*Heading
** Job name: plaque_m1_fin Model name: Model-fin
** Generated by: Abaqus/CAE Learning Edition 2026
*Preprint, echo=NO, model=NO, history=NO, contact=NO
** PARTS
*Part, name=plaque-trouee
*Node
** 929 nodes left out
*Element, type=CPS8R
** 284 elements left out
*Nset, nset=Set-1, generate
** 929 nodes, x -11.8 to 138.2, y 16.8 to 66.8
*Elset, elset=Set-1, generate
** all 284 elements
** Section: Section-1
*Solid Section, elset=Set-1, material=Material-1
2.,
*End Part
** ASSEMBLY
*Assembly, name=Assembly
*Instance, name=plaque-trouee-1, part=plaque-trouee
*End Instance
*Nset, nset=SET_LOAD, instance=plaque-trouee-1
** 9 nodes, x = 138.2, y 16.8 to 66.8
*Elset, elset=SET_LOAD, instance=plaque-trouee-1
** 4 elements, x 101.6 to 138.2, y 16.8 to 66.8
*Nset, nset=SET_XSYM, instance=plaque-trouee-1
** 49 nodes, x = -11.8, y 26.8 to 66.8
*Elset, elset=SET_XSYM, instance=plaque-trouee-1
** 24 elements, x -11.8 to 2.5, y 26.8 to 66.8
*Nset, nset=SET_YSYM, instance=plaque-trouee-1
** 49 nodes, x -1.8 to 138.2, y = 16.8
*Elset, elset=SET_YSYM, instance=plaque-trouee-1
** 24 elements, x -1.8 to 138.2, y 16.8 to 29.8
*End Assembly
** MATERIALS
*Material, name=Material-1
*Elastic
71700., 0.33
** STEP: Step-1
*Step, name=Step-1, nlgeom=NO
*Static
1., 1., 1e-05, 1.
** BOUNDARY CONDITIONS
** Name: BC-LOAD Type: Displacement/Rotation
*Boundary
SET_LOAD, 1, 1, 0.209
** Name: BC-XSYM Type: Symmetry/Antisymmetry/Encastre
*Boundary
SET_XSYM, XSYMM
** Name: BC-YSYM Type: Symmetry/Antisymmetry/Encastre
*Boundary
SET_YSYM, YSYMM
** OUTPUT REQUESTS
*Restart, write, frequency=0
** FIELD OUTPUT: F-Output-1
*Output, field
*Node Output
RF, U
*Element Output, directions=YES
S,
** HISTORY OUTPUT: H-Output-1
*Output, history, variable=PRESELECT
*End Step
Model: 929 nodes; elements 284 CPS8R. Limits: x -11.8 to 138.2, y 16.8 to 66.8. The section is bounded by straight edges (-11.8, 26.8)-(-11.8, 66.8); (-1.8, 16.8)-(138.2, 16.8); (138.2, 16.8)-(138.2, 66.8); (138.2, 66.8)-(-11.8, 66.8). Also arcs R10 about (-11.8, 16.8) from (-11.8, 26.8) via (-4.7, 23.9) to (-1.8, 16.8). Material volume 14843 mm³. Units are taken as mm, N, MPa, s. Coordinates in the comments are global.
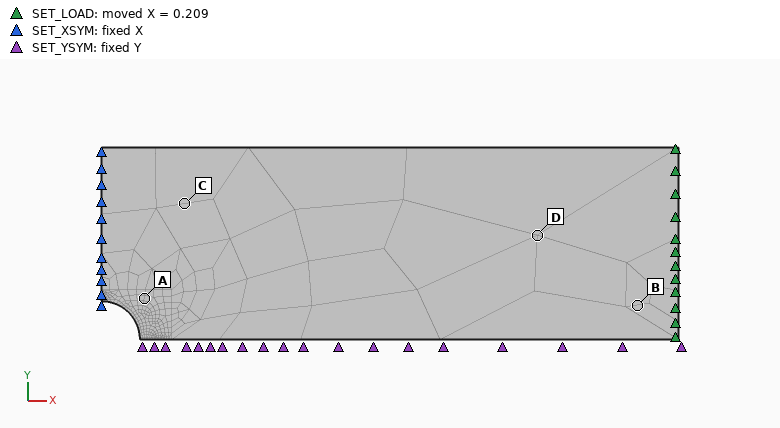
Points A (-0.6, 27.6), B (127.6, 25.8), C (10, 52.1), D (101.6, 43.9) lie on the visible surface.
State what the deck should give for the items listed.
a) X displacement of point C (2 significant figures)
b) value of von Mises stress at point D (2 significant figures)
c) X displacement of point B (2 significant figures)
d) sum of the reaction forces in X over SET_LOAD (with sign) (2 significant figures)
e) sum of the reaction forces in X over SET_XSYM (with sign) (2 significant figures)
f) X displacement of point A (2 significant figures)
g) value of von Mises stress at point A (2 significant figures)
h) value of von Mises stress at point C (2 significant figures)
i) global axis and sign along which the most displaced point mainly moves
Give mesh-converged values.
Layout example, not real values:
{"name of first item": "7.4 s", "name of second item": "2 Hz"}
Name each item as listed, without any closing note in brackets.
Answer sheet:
{"X displacement of point C": "0.032 mm", "value of von Mises stress at point D": "97 MPa", "X displacement of point B": "0.19 mm", "sum of the reaction forces in X over SET_LOAD (with sign)": "9700 N", "sum of the reaction forces in X over SET_XSYM (with sign)": "-9700 N", "X displacement of point A": "0.027 mm", "value of von Mises stress at point A": "130 MPa", "value of von Mises stress at point C": "110 MPa", "global axis and sign along which the most displaced point mainly moves": "+X"}
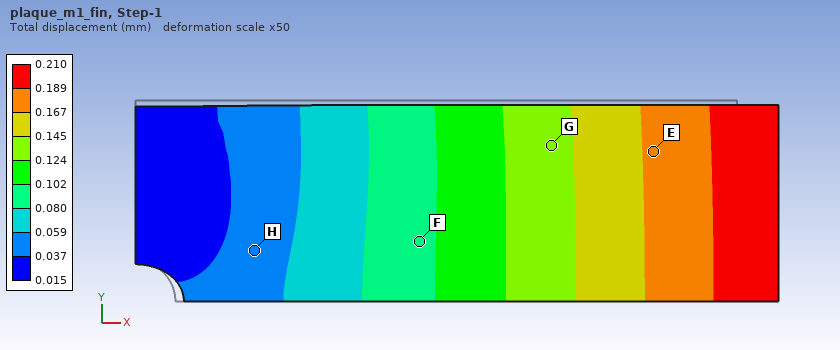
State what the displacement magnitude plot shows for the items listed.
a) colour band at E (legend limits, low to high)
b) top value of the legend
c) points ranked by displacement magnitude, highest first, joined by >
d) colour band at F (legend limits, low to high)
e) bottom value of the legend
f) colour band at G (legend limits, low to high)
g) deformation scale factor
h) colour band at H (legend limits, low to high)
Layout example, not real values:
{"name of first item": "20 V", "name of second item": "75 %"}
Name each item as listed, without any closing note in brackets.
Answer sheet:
{"colour band at E": "0.167 to 0.189 mm", "top value of the legend": "0.210 mm", "points ranked by displacement magnitude, highest first, joined by >": "E > G > F > H", "colour band at F": "0.080 to 0.102 mm", "bottom value of the legend": "0.015 mm", "colour band at G": "0.124 to 0.145 mm", "deformation scale factor": "50", "colour band at H": "0.037 to 0.059 mm"}
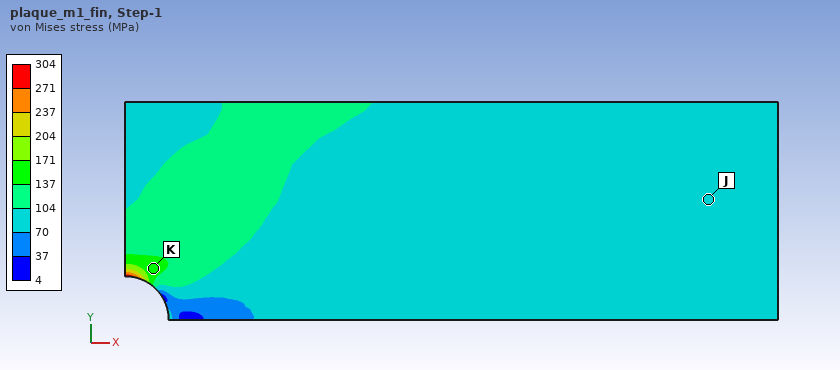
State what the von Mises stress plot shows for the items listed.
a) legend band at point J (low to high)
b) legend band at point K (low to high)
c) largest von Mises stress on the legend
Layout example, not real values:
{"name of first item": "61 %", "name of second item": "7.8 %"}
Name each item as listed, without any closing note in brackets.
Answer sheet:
{"legend band at point J": "70 to 104 MPa", "legend band at point K": "137 to 171 MPa", "largest von Mises stress on the legend": "304 MPa"}
